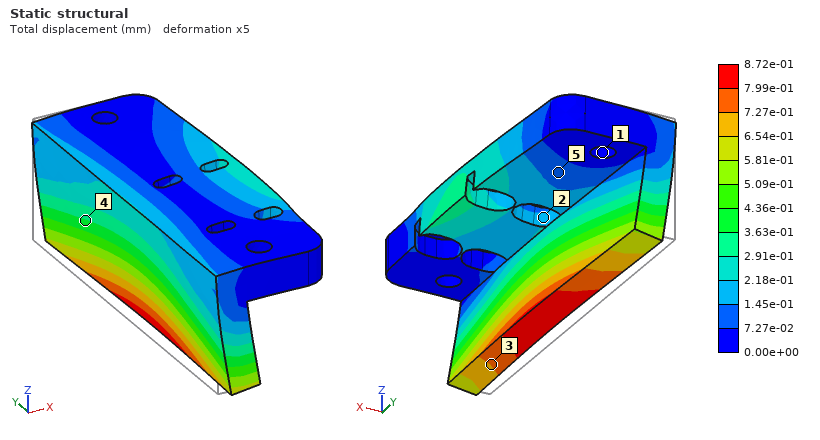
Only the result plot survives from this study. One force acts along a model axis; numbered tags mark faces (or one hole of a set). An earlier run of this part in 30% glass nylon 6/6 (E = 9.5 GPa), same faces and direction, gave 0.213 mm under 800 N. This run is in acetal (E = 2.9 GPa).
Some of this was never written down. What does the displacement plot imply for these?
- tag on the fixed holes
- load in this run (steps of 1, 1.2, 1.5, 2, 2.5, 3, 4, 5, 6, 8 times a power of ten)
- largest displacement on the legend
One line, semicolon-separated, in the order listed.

1; 1 kN; 8.72e-01 mm
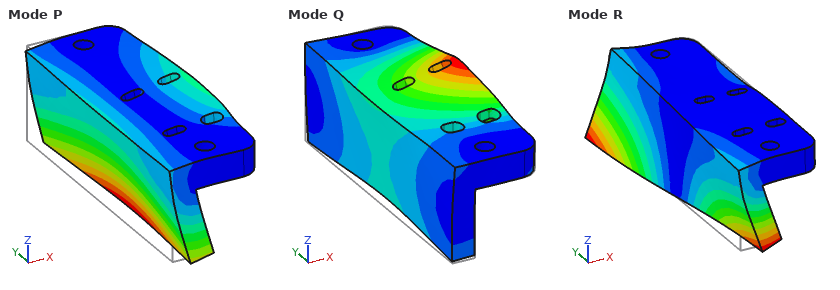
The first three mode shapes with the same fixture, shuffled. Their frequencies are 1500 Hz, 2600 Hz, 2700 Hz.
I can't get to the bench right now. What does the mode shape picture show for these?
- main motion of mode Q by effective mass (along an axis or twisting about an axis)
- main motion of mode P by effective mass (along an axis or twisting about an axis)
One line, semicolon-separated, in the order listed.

along Z; along X
